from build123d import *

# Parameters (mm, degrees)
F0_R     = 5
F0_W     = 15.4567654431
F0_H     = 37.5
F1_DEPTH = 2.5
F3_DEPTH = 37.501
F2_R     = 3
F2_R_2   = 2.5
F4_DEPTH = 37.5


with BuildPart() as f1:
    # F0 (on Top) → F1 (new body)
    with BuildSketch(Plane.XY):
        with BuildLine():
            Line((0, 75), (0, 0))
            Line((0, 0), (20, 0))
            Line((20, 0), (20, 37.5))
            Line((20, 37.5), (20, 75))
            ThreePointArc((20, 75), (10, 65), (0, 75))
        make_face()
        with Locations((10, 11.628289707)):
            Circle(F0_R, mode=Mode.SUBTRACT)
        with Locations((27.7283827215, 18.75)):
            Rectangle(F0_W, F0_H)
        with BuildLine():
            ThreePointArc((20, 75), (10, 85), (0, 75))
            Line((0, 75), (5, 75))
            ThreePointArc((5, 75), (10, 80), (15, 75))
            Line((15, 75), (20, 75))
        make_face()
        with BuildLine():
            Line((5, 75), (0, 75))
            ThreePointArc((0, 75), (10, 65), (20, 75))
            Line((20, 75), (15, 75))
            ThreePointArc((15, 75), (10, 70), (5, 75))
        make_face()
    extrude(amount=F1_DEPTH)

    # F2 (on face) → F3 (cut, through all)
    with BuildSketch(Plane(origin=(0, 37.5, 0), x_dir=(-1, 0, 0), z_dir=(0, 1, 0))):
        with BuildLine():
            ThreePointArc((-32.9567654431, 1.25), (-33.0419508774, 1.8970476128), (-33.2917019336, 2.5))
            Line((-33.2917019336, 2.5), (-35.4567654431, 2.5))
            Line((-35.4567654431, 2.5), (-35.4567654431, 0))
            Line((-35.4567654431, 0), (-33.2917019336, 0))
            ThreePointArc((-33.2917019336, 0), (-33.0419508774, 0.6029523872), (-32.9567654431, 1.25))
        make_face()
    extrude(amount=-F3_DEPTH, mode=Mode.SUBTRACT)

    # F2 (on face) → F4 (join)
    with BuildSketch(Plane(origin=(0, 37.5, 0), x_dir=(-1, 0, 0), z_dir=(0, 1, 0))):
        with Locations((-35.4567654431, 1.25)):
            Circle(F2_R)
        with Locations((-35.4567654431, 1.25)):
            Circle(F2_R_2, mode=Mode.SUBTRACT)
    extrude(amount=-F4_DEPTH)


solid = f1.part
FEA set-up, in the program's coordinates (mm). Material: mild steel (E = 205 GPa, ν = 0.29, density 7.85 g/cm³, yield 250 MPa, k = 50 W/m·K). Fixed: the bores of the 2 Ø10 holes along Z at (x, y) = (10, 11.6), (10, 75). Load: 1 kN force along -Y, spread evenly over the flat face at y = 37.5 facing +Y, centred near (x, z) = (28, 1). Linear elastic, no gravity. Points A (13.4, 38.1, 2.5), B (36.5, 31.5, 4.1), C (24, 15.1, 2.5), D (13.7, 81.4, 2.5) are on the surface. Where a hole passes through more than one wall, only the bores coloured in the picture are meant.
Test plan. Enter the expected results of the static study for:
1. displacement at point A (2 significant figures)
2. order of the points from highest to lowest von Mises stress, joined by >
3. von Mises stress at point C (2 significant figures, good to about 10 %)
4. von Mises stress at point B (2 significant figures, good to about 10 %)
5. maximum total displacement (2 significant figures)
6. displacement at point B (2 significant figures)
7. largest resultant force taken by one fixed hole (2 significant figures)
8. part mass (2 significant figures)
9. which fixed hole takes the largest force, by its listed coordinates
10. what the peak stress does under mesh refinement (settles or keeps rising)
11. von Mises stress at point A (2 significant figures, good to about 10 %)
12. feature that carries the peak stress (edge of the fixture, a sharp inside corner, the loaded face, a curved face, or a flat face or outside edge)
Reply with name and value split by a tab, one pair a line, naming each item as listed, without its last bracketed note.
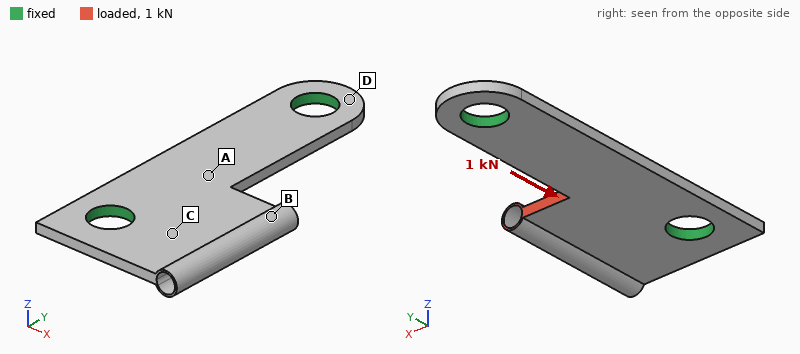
displacement at point A	3.5 µm
order of the points from highest to lowest von Mises stress, joined by >	B > C > A > D
von Mises stress at point C	18 MPa
von Mises stress at point B	24 MPa
maximum total displacement	9.9 µm
displacement at point B	8.0 µm
largest resultant force taken by one fixed hole	810 N
part mass	41 g
which fixed hole takes the largest force, by its listed coordinates	(10, 11.6)
what the peak stress does under mesh refinement	keeps rising
von Mises stress at point A	11 MPa
feature that carries the peak stress	a sharp inside corner
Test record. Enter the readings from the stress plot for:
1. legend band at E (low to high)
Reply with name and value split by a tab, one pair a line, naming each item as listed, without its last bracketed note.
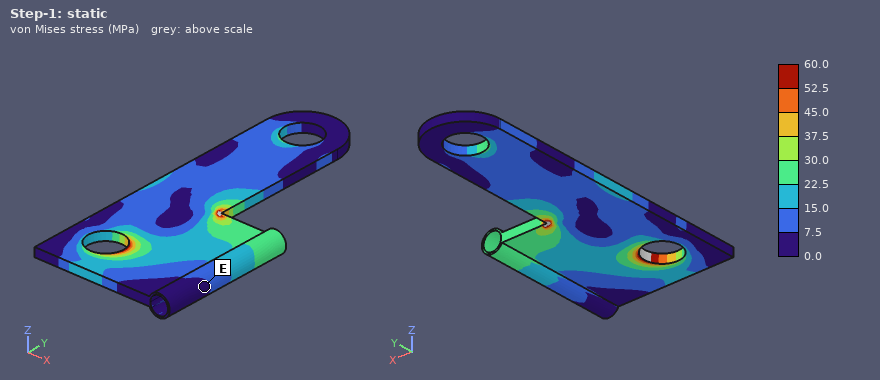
legend band at E	0.0 to 7.5 MPa
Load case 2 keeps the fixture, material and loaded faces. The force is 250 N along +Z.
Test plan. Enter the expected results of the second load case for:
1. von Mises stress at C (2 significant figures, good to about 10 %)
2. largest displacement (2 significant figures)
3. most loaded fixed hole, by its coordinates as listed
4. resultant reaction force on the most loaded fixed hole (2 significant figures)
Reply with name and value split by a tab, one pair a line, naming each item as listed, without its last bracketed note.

von Mises stress at C	74 MPa
largest displacement	0.18 mm
most loaded fixed hole, by its coordinates as listed	(10, 11.6)
resultant reaction force on the most loaded fixed hole	190 N
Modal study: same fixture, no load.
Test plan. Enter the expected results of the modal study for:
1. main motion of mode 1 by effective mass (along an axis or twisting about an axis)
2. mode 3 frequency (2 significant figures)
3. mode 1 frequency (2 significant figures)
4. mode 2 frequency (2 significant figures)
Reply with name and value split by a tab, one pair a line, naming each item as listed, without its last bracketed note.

main motion of mode 1 by effective mass	along Z
mode 3 frequency	6100 Hz
mode 1 frequency	3100 Hz
mode 2 frequency	4300 Hz
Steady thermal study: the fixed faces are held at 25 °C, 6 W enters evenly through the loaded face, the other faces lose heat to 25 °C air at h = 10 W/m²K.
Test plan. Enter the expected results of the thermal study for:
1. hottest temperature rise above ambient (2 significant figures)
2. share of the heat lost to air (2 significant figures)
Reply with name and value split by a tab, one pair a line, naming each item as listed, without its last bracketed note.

hottest temperature rise above ambient	55 K
share of the heat lost to air	11 %
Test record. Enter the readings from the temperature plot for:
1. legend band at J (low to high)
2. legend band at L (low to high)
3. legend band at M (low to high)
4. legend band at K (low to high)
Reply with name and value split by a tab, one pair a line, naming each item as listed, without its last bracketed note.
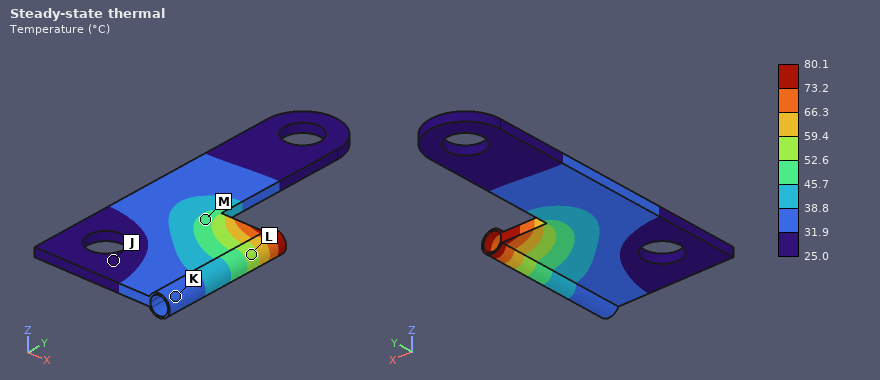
legend band at J	25.0 to 31.9 °C
legend band at L	52.6 to 59.4 °C
legend band at M	45.7 to 52.6 °C
legend band at K	31.9 to 38.8 °C
